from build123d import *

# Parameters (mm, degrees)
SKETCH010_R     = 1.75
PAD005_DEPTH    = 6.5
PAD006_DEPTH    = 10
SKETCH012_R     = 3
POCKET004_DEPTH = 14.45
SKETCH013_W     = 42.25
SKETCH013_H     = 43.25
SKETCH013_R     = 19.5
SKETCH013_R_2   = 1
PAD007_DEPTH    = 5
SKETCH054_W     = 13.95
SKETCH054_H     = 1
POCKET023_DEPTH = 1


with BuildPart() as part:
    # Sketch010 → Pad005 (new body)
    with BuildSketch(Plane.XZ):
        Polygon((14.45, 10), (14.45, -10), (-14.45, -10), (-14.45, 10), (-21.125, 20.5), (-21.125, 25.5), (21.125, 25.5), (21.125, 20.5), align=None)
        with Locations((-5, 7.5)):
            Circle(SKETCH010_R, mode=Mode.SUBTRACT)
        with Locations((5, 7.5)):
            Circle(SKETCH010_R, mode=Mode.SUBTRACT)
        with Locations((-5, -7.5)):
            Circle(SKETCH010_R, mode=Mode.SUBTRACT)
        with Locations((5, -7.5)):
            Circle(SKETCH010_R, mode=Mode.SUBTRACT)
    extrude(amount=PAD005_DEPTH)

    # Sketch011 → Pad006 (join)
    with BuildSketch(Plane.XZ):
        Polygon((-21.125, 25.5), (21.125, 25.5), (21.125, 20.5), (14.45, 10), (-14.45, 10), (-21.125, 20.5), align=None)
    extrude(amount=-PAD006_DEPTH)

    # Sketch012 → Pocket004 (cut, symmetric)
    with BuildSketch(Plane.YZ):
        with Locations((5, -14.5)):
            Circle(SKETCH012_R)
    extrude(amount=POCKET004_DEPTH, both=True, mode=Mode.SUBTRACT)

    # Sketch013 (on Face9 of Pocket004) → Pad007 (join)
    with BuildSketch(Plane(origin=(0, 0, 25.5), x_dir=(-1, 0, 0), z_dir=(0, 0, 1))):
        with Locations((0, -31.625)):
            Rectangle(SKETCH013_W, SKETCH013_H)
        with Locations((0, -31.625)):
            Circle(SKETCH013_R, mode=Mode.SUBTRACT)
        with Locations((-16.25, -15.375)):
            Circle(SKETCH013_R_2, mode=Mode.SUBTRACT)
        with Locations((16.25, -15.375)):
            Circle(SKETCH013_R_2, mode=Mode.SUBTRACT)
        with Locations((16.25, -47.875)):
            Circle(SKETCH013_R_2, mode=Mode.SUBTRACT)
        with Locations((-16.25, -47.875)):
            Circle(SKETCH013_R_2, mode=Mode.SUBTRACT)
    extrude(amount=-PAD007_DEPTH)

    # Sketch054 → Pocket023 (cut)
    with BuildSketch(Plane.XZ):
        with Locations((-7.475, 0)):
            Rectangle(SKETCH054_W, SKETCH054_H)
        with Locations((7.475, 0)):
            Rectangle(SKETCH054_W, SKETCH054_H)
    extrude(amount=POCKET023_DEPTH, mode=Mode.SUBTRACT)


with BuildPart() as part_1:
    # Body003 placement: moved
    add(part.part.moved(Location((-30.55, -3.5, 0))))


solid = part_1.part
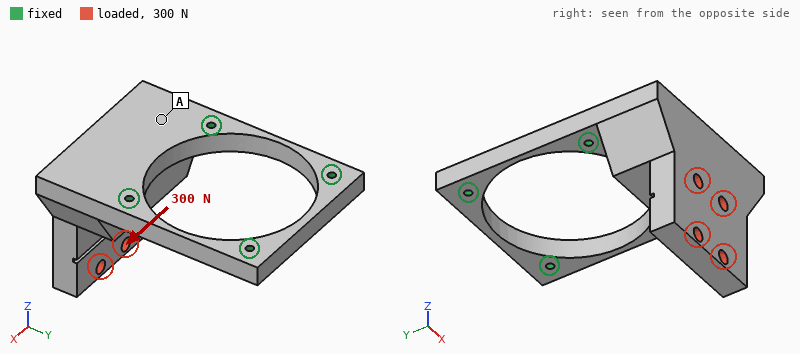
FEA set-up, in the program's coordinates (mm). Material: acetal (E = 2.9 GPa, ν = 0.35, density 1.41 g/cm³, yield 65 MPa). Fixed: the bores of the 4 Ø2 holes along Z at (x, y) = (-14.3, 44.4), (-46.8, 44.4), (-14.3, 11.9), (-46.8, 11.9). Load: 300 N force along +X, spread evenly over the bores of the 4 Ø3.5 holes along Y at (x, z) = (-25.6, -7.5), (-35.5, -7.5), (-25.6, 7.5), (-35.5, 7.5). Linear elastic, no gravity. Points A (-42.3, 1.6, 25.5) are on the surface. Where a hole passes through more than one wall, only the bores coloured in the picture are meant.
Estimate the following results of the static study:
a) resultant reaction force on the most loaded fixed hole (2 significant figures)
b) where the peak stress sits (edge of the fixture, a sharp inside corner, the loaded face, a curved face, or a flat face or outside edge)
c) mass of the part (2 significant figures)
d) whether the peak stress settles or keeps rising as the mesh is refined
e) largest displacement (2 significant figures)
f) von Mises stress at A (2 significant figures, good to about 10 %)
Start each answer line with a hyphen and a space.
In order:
- 300 N
- edge of the fixture
- 23 g
- keeps rising
- 0.29 mm
- 3.3 MPa
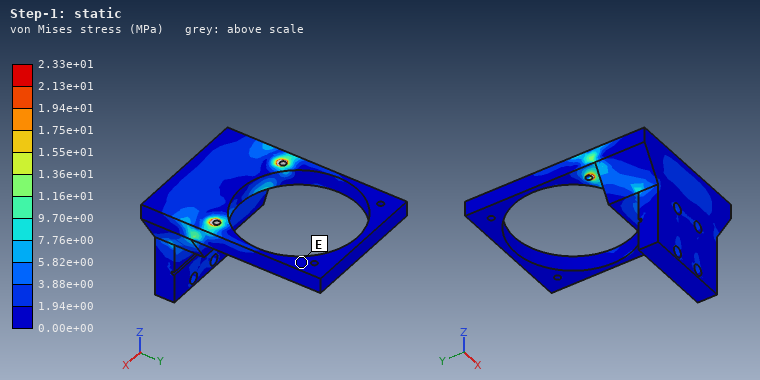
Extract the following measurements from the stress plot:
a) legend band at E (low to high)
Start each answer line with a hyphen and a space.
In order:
- 0.00e+00 to 1.94e+00 MPa
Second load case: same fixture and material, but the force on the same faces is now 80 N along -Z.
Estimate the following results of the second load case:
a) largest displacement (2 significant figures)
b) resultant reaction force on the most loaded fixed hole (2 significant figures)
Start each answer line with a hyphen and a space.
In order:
- 0.61 mm
- 42 N
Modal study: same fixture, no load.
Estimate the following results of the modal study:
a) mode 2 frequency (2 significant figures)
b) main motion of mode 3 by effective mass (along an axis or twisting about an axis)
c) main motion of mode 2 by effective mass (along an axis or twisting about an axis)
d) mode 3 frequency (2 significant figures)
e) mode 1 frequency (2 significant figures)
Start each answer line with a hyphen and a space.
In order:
- 2200 Hz
- along Z
- along X
- 2700 Hz
- 550 Hz
